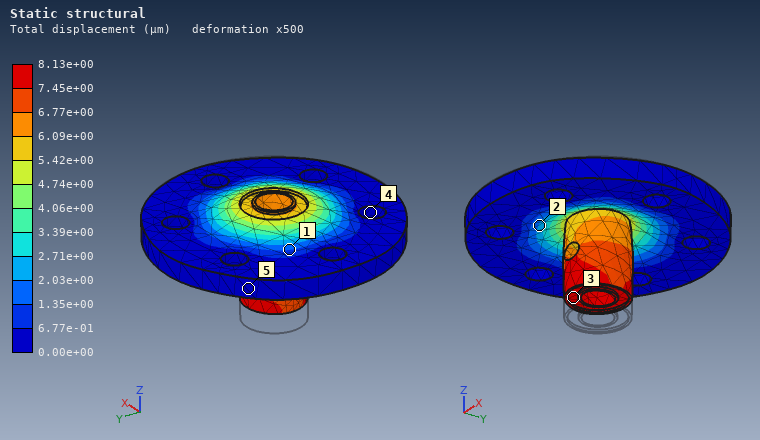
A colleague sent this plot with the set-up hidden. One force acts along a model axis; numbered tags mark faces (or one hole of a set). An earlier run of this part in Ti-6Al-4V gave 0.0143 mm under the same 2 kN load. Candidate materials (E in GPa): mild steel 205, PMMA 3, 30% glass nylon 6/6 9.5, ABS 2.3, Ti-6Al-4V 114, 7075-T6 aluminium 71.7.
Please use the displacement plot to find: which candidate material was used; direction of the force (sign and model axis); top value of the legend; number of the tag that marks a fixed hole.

mild steel
+Z
8.13e+00 µm
4
